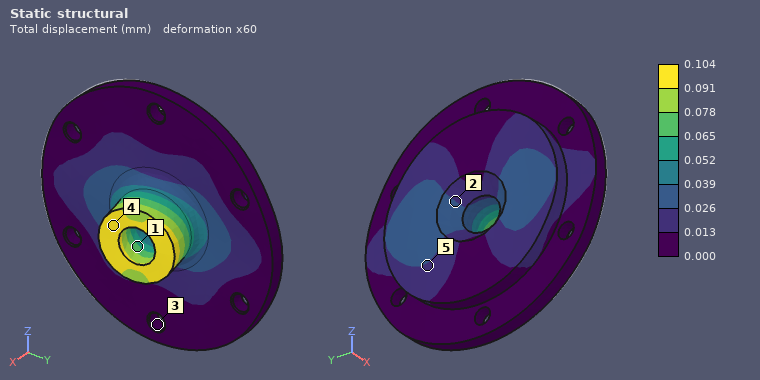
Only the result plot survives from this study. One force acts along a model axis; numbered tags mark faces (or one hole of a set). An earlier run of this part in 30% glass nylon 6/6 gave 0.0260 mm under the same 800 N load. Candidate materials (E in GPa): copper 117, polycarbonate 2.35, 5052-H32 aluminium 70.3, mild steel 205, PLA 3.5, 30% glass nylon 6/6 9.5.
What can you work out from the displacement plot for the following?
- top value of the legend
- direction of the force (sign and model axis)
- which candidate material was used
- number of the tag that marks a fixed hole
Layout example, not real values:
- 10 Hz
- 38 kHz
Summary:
- 0.104 mm
- +Y
- polycarbonate
- 3
